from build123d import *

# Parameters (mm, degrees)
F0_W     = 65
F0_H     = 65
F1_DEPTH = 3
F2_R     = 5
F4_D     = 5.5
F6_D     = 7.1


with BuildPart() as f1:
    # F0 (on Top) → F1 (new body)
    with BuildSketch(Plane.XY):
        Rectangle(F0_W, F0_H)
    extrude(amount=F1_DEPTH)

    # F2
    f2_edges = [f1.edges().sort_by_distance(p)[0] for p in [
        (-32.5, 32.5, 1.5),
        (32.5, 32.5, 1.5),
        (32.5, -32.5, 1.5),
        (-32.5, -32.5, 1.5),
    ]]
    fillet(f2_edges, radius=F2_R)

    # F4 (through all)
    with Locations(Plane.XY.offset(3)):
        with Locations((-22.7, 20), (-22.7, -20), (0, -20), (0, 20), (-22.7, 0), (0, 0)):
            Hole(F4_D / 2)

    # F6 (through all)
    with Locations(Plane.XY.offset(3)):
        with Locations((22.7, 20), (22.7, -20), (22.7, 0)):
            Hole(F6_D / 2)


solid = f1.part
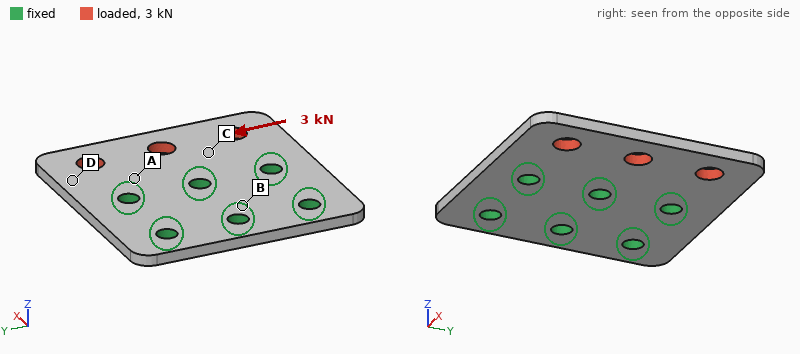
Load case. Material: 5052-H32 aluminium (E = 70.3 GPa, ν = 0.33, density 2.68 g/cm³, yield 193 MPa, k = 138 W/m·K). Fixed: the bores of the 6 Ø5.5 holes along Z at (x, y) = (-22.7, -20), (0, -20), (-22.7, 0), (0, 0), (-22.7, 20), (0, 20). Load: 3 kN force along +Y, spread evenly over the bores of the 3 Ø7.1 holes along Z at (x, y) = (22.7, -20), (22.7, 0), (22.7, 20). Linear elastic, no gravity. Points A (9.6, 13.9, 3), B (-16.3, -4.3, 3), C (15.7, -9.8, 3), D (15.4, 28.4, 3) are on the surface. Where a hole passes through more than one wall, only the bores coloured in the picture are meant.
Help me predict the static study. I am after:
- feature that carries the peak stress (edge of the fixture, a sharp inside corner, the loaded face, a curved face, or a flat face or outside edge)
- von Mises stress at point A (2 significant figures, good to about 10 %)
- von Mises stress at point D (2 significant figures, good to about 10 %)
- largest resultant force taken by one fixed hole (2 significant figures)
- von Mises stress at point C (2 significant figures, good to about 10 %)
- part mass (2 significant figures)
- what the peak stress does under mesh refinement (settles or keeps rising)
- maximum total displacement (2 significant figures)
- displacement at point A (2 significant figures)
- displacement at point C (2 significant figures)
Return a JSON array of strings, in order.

["edge of the fixture", "37 MPa", "14 MPa", "1.5 kN", "32 MPa", "32 g", "keeps rising", "27 µm", "7.1 µm", "12 µm"]
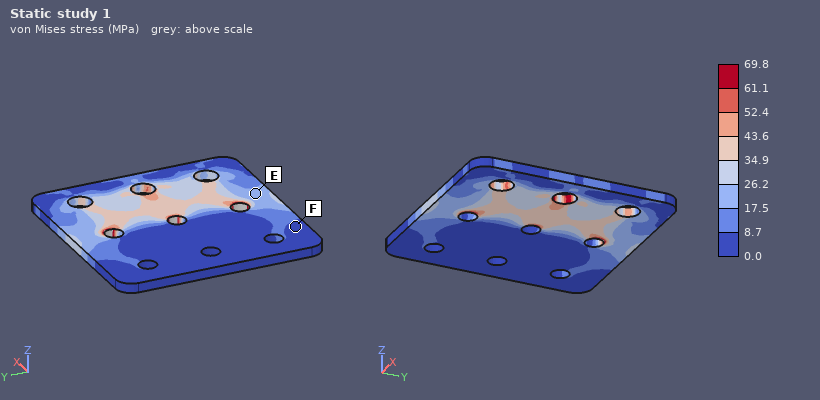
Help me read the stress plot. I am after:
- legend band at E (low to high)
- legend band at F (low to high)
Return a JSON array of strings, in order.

["17.5 to 26.2 MPa", "0.0 to 8.7 MPa"]
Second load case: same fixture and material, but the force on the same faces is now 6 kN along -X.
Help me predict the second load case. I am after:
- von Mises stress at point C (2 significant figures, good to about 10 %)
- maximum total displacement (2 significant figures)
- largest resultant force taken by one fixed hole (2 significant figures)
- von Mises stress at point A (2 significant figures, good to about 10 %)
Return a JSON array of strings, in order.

["30 MPa", "16 µm", "1.8 kN", "32 MPa"]
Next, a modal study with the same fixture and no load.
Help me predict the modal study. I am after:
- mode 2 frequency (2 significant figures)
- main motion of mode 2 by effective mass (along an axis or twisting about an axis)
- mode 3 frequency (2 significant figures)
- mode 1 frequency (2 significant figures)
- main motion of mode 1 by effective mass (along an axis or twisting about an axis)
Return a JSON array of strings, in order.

["3800 Hz", "twisting about X", "6500 Hz", "2700 Hz", "along Z"]
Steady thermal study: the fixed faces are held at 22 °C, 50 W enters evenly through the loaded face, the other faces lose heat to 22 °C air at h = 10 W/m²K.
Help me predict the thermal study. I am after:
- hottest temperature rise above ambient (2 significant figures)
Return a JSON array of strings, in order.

["51 K"]
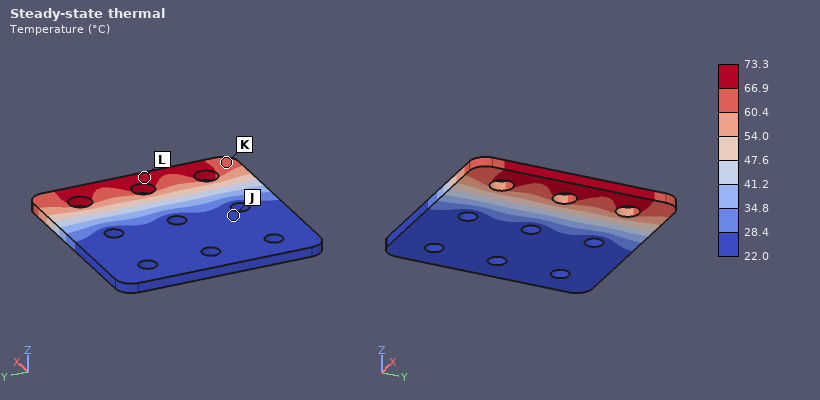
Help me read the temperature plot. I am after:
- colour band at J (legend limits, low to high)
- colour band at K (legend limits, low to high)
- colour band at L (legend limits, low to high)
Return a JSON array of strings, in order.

["22.0 to 28.4 °C", "60.4 to 66.9 °C", "66.9 to 73.3 °C"]
